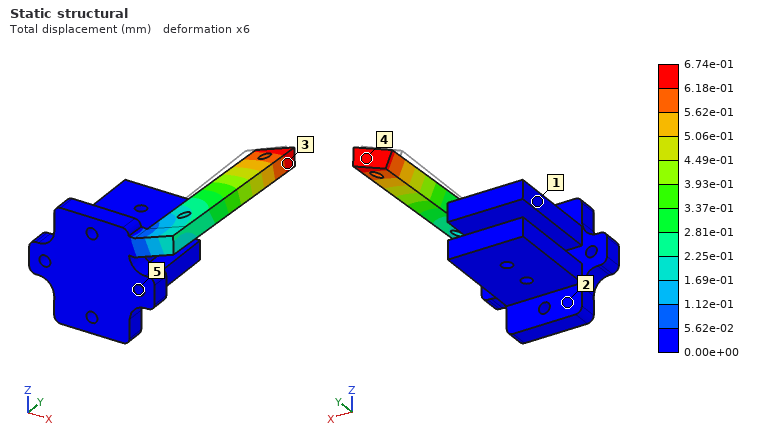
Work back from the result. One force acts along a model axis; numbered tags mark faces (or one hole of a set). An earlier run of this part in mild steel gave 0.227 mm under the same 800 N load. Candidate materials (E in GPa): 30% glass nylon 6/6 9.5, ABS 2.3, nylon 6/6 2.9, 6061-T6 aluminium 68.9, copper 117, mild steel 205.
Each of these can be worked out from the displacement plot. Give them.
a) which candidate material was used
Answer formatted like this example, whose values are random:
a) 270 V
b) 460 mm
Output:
a) 6061-T6 aluminium
